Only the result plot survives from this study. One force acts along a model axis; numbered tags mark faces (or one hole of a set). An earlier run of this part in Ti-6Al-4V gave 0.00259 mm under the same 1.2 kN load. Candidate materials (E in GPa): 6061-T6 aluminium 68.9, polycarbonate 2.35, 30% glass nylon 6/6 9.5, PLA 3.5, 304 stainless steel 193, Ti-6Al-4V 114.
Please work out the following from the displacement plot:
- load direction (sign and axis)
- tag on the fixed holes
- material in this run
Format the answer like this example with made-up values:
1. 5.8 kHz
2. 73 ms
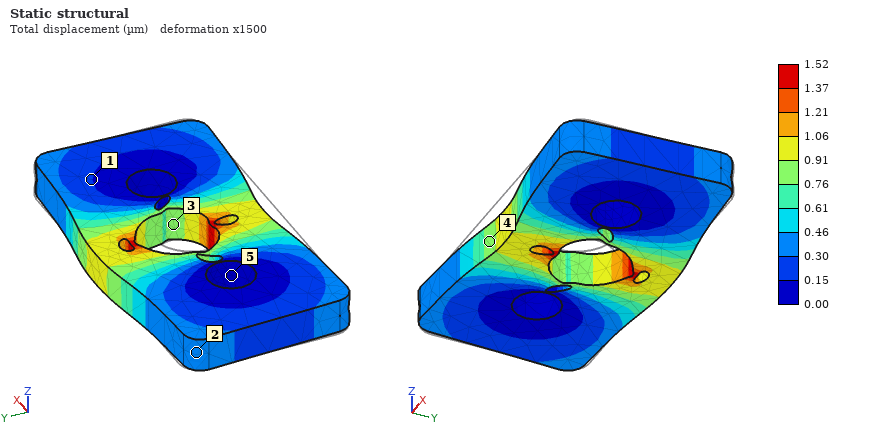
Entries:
1. +Y
2. 5
3. 304 stainless steel
